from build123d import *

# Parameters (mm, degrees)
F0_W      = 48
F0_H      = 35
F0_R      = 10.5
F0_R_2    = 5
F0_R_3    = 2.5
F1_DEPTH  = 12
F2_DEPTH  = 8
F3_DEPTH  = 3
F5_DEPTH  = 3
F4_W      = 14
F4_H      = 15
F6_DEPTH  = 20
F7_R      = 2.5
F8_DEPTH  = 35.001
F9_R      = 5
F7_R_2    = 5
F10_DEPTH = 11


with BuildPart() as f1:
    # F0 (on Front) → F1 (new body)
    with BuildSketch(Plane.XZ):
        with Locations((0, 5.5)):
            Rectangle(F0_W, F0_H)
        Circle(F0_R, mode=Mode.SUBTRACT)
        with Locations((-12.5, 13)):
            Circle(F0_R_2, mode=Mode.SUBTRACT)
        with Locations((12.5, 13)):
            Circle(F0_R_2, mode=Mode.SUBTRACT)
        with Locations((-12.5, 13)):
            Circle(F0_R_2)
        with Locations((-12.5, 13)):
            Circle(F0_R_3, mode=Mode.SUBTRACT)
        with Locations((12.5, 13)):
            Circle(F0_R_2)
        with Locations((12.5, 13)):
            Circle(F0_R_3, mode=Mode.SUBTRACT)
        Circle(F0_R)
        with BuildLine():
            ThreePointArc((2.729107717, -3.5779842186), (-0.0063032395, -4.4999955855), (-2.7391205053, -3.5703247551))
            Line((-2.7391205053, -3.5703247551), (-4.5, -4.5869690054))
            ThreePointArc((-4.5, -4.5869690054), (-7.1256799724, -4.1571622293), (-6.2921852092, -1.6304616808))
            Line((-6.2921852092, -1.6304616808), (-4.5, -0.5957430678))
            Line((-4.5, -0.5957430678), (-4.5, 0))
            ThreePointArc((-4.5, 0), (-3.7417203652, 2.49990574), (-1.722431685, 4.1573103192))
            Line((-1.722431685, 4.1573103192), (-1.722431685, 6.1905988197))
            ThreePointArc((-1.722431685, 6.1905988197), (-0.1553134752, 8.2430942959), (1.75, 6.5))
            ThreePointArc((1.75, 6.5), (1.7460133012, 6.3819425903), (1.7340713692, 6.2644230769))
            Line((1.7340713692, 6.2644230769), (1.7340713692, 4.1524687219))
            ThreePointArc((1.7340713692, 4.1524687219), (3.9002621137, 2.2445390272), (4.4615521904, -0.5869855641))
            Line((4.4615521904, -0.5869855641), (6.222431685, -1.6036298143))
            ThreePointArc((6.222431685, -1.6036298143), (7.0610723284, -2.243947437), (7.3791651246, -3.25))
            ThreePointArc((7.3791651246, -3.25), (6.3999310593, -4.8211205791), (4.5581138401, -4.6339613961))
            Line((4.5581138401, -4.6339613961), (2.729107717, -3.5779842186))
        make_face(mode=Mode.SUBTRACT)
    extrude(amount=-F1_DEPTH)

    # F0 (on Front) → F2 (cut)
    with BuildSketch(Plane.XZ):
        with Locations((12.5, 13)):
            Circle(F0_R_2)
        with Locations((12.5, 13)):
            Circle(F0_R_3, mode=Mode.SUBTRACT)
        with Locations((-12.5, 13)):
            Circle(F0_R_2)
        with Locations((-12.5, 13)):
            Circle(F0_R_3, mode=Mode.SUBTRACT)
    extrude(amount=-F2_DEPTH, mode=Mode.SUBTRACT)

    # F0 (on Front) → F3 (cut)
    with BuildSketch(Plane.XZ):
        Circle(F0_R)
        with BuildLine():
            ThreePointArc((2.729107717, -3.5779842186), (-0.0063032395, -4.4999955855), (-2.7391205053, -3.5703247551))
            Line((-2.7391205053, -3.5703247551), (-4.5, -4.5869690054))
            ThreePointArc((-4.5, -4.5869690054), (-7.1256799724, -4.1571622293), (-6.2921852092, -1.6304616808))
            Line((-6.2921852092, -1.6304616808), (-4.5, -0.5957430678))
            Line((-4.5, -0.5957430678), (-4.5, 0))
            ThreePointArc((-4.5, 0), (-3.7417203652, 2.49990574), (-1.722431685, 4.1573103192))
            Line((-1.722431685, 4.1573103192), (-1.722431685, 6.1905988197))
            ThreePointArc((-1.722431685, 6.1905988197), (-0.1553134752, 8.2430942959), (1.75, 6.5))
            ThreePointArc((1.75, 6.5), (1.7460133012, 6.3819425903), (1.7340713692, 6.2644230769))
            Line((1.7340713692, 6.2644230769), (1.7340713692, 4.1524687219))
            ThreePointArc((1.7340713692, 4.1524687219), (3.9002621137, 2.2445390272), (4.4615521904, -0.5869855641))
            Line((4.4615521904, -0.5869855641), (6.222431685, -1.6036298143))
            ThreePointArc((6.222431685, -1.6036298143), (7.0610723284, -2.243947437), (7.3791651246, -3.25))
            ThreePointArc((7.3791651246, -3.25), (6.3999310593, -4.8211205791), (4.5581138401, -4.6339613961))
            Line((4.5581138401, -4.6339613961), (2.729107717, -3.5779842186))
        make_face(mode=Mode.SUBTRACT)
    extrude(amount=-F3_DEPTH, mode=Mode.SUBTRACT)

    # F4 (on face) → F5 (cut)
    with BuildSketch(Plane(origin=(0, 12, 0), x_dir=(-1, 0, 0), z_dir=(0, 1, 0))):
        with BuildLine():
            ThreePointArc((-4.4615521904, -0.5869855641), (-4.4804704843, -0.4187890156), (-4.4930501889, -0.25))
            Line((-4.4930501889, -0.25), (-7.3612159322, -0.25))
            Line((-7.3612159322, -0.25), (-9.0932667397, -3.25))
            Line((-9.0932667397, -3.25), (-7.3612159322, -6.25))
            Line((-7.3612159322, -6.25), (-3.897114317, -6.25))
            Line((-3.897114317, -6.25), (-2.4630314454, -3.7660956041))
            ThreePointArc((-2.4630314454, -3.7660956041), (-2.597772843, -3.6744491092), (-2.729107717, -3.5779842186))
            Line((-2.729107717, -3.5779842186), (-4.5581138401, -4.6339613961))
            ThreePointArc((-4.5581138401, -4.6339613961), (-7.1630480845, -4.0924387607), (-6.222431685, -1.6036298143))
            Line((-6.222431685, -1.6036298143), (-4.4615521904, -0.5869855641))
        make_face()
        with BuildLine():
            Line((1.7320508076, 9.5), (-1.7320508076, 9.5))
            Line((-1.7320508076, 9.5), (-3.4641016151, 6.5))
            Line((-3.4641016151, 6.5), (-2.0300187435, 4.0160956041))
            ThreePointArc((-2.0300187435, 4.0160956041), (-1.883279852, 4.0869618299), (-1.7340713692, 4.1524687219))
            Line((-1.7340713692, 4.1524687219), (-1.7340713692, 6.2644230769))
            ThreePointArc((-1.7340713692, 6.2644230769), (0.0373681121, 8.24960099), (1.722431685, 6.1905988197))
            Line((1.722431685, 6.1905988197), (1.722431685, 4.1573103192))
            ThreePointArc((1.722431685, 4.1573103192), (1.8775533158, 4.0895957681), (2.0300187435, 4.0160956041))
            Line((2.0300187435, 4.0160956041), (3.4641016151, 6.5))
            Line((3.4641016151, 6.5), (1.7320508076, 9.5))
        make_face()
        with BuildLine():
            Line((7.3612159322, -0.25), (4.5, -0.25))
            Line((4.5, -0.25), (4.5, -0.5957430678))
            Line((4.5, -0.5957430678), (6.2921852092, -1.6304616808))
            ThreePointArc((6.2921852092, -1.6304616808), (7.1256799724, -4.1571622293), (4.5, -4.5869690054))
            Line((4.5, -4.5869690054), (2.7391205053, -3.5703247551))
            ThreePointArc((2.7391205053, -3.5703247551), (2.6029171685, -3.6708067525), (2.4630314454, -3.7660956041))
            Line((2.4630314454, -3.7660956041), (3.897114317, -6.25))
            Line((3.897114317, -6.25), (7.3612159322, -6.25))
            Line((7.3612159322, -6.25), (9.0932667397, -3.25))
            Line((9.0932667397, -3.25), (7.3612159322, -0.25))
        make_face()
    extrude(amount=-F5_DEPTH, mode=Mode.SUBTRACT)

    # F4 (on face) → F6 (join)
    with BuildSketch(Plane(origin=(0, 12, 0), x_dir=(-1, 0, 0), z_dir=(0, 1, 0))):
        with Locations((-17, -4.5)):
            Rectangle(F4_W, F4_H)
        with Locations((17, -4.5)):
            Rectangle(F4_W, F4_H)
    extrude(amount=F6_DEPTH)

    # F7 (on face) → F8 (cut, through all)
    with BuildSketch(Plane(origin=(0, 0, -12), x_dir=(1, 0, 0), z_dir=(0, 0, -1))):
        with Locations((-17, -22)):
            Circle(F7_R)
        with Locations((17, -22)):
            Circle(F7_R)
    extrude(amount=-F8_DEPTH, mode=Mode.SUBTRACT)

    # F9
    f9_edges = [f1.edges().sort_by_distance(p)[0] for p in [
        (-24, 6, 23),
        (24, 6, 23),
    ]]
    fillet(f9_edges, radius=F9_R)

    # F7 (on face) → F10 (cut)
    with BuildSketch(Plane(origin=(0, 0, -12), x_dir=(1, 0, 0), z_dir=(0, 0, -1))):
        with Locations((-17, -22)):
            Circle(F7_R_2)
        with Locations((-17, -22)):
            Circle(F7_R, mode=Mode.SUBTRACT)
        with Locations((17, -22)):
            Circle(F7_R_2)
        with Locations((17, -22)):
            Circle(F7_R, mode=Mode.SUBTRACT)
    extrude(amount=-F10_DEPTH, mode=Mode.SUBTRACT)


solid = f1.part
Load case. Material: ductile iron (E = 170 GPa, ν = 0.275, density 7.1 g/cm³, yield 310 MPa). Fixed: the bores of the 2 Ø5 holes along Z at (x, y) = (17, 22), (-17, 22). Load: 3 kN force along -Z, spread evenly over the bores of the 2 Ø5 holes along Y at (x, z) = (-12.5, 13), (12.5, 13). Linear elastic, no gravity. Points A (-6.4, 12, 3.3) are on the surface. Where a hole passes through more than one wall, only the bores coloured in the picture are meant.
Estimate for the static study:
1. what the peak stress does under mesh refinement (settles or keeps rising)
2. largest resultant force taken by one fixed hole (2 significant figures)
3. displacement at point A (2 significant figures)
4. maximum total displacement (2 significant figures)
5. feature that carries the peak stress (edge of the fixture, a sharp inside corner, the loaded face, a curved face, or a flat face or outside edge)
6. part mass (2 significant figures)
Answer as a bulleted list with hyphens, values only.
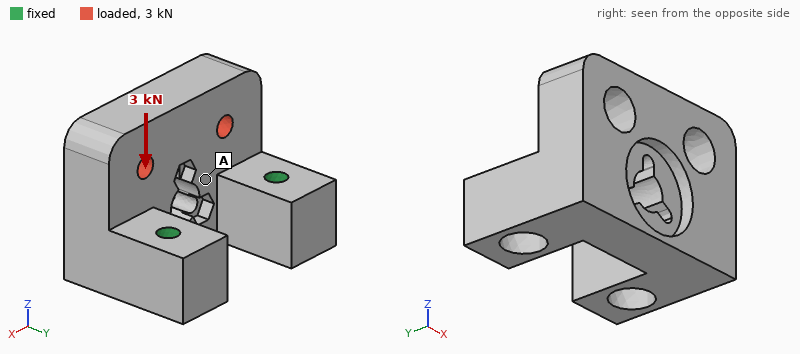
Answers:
- keeps rising
- 1.5 kN
- 18 µm
- 48 µm
- edge of the fixture
- 160 g
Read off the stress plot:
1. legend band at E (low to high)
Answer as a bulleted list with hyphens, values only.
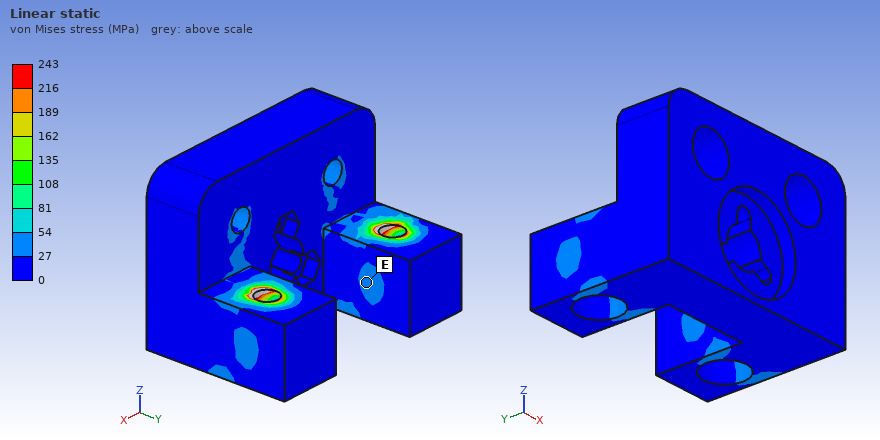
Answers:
- 27 to 54 MPa
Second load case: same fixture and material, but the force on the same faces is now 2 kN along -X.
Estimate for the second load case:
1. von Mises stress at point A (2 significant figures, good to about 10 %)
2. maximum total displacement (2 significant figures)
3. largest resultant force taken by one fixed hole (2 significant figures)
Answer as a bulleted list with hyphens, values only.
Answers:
- 26 MPa
- 15 µm
- 1.2 kN
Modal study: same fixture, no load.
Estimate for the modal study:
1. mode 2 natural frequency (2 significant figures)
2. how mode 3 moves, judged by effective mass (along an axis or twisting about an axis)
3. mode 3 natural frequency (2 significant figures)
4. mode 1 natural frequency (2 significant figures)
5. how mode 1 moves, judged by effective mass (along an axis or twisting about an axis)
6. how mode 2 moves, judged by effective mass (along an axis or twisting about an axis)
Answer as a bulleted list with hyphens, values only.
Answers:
- 6600 Hz
- along X
- 9300 Hz
- 3200 Hz
- along Z
- along X
